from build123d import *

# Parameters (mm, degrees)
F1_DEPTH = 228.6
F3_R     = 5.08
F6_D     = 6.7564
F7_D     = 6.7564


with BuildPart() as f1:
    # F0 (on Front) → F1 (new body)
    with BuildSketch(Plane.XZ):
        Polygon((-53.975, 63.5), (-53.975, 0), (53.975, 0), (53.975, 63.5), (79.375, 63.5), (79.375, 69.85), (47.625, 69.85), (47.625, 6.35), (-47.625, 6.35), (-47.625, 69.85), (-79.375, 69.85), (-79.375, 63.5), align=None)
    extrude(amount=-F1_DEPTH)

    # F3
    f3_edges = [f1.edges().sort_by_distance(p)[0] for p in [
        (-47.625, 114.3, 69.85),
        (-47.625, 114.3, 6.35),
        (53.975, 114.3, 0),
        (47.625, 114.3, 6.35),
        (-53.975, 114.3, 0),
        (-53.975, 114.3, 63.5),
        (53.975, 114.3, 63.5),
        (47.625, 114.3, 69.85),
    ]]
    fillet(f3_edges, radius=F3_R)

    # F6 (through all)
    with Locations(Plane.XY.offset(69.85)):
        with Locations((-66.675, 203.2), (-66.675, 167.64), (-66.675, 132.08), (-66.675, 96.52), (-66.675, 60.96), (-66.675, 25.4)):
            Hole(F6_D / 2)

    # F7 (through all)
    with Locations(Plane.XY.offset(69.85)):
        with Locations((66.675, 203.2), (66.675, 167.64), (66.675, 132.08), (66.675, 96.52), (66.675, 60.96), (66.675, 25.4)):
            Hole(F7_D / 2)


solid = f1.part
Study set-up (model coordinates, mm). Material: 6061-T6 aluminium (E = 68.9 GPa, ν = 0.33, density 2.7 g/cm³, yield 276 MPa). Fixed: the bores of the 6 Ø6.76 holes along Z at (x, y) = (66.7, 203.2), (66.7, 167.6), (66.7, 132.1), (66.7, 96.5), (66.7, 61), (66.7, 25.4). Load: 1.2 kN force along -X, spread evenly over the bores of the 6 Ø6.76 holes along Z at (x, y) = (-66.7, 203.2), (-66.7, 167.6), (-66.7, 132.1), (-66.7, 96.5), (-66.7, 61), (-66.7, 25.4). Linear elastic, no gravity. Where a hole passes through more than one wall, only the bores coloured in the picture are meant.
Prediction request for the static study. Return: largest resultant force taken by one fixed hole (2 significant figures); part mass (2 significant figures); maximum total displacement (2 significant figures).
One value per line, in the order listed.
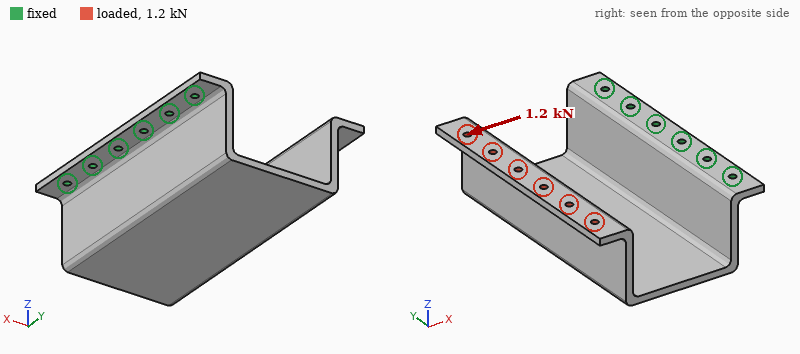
270 N
1.1 kg
3.1 mm
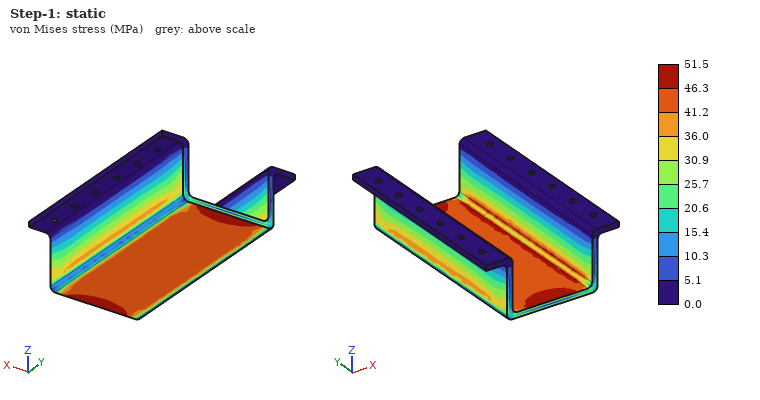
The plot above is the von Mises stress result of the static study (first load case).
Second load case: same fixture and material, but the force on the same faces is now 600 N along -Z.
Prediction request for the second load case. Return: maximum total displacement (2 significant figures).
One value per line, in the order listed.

3.0 mm
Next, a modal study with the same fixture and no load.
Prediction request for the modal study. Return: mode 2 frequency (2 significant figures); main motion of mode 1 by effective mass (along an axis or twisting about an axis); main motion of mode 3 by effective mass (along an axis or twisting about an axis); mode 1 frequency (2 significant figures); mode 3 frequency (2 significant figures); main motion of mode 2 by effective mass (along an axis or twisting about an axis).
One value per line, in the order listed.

220 Hz
along Z
along X
120 Hz
330 Hz
along Y
